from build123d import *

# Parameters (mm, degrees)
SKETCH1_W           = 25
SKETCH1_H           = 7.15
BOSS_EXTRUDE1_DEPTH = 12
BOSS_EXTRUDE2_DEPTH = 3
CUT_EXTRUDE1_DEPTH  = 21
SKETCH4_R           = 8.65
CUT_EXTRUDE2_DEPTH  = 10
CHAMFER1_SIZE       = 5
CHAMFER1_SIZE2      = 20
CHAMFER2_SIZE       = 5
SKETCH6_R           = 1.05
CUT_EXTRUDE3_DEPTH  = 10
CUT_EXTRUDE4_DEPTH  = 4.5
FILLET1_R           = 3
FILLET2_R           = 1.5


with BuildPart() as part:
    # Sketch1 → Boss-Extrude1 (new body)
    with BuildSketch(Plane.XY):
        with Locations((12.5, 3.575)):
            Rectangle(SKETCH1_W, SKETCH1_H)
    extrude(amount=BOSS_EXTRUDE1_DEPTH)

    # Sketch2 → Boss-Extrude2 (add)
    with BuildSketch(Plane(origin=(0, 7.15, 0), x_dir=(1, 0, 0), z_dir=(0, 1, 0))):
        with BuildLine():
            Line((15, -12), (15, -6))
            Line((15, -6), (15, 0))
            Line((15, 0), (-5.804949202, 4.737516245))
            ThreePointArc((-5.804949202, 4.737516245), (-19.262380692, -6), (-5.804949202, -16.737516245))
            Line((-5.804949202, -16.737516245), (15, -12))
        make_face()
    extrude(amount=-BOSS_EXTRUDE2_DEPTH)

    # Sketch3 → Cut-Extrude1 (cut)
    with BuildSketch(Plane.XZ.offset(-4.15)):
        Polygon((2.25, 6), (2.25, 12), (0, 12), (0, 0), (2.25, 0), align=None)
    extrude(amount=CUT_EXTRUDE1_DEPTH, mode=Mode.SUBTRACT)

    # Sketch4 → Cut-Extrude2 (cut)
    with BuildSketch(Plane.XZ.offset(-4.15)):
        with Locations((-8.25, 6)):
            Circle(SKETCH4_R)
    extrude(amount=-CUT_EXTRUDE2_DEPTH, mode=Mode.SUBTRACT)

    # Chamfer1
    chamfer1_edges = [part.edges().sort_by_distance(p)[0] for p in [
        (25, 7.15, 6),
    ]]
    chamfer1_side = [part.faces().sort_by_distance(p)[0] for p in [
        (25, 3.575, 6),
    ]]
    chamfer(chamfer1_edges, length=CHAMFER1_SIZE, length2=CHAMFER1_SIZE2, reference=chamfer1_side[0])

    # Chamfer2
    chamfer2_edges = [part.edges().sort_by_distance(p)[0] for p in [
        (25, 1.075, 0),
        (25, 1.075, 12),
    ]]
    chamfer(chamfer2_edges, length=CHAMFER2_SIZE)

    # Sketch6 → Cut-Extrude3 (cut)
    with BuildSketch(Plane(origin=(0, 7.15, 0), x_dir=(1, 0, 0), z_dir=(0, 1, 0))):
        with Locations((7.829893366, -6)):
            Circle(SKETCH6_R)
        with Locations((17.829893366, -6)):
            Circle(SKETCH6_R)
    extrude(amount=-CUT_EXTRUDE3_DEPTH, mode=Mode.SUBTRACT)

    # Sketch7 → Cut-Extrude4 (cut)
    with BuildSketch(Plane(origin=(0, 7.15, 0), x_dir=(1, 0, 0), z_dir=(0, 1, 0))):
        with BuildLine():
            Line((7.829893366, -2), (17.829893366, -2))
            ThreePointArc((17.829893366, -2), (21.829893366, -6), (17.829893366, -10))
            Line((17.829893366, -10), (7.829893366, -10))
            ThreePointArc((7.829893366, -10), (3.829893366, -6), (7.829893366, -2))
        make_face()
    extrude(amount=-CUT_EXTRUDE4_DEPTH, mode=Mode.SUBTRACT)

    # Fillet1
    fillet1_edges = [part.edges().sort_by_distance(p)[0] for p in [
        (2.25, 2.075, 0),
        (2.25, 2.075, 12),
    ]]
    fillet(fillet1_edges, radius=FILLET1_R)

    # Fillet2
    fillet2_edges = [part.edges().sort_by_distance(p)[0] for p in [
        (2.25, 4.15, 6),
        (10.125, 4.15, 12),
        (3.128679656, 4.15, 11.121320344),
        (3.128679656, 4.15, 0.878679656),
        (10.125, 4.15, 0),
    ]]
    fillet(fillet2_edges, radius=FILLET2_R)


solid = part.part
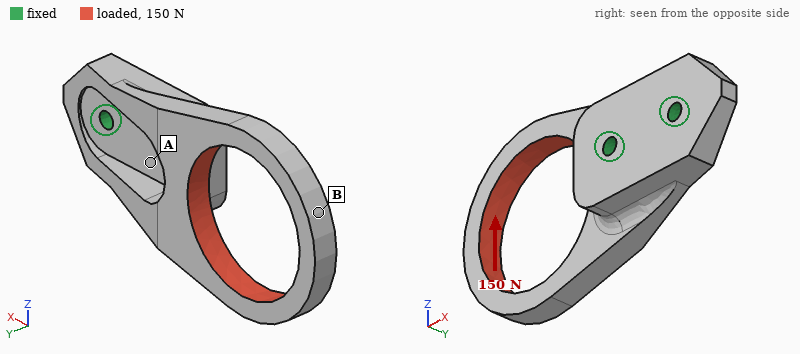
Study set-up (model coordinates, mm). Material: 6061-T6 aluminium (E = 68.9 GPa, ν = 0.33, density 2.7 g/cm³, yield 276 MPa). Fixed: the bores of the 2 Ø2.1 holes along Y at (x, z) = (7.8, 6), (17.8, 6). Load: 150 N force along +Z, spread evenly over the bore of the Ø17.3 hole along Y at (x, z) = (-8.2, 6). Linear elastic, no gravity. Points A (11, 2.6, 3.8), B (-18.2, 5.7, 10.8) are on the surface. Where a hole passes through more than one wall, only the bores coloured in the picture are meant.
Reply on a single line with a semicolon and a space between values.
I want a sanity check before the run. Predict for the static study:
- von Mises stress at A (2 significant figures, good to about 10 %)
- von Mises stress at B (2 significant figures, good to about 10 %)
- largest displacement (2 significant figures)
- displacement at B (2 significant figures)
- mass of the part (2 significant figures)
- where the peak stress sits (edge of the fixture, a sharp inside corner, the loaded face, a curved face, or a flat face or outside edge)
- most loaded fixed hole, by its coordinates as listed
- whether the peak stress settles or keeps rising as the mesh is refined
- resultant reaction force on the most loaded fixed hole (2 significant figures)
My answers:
11 MPa; 29 MPa; 75 µm; 73 µm; 4.1 g; edge of the fixture; (7.8, 6); keeps rising; 340 N
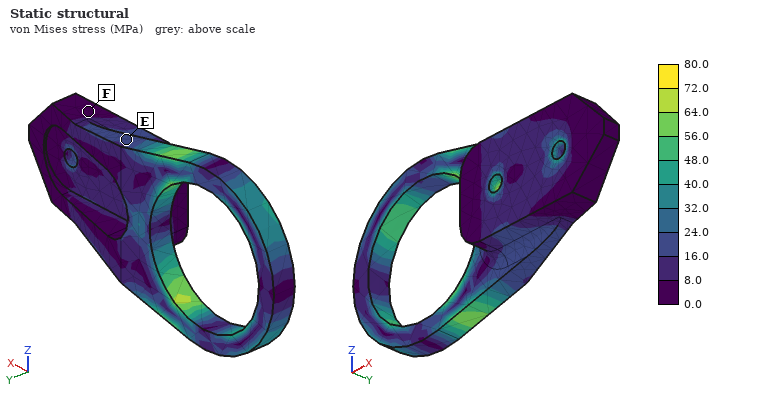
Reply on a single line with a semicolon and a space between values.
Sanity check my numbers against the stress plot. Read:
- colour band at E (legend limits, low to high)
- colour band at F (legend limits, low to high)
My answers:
16.0 to 24.0 MPa; 0.0 to 8.0 MPa
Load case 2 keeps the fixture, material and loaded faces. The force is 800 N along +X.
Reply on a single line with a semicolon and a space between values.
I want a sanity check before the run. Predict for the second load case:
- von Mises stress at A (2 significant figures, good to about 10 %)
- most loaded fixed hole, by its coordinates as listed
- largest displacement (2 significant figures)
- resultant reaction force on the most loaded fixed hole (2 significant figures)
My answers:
32 MPa; (17.8, 6); 78 µm; 510 N
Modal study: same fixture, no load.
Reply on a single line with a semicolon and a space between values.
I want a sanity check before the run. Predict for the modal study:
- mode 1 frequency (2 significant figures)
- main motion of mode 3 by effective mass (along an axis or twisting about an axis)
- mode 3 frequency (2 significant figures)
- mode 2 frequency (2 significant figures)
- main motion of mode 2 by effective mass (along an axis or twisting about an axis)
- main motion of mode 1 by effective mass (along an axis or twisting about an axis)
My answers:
4000 Hz; twisting about X; 7900 Hz; 7200 Hz; along Z; along Y
